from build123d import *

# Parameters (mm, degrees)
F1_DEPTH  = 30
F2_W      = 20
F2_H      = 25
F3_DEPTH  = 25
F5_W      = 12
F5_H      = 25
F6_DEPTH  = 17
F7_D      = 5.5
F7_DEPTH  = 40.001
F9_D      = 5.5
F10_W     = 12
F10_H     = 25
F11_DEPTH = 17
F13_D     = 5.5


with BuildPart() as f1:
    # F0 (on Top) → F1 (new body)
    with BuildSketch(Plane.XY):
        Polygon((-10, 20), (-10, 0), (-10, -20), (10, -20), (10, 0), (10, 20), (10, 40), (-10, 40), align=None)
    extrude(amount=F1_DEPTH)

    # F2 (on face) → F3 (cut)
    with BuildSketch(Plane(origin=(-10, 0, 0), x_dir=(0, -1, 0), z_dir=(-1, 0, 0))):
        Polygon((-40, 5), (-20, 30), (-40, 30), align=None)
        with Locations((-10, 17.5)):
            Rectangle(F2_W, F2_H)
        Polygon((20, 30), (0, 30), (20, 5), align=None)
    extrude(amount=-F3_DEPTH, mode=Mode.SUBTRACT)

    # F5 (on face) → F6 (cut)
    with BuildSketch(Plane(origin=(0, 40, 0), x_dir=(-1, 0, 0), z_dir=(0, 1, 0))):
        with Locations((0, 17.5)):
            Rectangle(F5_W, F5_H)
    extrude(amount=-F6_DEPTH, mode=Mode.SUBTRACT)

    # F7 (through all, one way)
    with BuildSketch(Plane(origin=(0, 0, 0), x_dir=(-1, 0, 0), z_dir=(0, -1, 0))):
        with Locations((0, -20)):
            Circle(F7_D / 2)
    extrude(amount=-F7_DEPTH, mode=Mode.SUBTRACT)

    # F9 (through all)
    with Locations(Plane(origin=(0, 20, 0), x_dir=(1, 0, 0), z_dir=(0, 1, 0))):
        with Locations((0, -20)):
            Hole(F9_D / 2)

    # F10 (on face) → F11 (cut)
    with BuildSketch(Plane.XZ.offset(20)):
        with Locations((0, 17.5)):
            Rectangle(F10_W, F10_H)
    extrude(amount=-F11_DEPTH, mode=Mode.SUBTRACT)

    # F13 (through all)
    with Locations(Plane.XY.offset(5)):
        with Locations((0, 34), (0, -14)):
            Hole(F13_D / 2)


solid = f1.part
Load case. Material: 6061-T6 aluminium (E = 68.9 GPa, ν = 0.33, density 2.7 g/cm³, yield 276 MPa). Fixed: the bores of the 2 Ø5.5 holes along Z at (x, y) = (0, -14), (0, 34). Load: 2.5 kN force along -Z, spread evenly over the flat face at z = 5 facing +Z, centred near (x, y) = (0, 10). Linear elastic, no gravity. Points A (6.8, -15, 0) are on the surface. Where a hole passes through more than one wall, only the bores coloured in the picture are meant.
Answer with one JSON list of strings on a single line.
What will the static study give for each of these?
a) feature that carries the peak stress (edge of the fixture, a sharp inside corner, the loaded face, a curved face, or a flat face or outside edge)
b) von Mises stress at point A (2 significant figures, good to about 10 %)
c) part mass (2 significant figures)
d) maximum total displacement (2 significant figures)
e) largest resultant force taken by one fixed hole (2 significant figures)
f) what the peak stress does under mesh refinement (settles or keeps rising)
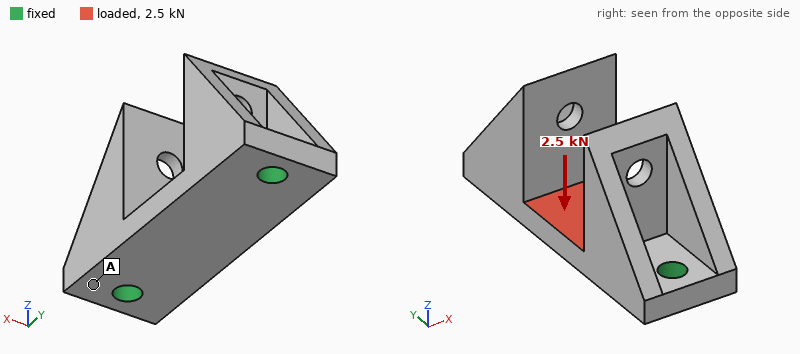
["edge of the fixture", "42 MPa", "30 g", "92 µm", "1.3 kN", "keeps rising"]
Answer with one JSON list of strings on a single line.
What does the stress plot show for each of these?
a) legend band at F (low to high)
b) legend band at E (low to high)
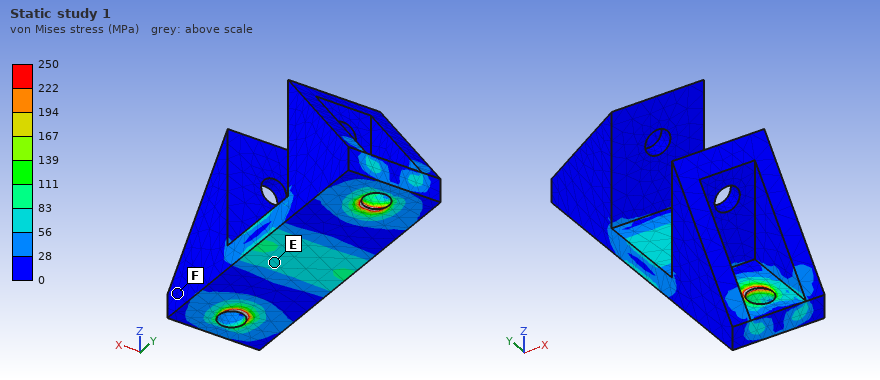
["0 to 28 MPa", "56 to 83 MPa"]
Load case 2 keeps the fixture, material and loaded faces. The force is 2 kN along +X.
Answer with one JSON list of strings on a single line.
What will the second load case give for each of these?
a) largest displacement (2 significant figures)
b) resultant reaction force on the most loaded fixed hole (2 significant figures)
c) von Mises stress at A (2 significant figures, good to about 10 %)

["29 µm", "1.0 kN", "16 MPa"]
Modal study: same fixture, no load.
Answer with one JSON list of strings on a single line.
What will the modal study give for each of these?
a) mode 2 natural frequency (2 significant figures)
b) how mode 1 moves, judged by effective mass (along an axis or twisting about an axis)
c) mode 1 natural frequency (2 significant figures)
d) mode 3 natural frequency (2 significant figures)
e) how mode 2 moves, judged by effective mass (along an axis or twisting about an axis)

["7300 Hz", "along X", "6800 Hz", "8800 Hz", "along Z"]
